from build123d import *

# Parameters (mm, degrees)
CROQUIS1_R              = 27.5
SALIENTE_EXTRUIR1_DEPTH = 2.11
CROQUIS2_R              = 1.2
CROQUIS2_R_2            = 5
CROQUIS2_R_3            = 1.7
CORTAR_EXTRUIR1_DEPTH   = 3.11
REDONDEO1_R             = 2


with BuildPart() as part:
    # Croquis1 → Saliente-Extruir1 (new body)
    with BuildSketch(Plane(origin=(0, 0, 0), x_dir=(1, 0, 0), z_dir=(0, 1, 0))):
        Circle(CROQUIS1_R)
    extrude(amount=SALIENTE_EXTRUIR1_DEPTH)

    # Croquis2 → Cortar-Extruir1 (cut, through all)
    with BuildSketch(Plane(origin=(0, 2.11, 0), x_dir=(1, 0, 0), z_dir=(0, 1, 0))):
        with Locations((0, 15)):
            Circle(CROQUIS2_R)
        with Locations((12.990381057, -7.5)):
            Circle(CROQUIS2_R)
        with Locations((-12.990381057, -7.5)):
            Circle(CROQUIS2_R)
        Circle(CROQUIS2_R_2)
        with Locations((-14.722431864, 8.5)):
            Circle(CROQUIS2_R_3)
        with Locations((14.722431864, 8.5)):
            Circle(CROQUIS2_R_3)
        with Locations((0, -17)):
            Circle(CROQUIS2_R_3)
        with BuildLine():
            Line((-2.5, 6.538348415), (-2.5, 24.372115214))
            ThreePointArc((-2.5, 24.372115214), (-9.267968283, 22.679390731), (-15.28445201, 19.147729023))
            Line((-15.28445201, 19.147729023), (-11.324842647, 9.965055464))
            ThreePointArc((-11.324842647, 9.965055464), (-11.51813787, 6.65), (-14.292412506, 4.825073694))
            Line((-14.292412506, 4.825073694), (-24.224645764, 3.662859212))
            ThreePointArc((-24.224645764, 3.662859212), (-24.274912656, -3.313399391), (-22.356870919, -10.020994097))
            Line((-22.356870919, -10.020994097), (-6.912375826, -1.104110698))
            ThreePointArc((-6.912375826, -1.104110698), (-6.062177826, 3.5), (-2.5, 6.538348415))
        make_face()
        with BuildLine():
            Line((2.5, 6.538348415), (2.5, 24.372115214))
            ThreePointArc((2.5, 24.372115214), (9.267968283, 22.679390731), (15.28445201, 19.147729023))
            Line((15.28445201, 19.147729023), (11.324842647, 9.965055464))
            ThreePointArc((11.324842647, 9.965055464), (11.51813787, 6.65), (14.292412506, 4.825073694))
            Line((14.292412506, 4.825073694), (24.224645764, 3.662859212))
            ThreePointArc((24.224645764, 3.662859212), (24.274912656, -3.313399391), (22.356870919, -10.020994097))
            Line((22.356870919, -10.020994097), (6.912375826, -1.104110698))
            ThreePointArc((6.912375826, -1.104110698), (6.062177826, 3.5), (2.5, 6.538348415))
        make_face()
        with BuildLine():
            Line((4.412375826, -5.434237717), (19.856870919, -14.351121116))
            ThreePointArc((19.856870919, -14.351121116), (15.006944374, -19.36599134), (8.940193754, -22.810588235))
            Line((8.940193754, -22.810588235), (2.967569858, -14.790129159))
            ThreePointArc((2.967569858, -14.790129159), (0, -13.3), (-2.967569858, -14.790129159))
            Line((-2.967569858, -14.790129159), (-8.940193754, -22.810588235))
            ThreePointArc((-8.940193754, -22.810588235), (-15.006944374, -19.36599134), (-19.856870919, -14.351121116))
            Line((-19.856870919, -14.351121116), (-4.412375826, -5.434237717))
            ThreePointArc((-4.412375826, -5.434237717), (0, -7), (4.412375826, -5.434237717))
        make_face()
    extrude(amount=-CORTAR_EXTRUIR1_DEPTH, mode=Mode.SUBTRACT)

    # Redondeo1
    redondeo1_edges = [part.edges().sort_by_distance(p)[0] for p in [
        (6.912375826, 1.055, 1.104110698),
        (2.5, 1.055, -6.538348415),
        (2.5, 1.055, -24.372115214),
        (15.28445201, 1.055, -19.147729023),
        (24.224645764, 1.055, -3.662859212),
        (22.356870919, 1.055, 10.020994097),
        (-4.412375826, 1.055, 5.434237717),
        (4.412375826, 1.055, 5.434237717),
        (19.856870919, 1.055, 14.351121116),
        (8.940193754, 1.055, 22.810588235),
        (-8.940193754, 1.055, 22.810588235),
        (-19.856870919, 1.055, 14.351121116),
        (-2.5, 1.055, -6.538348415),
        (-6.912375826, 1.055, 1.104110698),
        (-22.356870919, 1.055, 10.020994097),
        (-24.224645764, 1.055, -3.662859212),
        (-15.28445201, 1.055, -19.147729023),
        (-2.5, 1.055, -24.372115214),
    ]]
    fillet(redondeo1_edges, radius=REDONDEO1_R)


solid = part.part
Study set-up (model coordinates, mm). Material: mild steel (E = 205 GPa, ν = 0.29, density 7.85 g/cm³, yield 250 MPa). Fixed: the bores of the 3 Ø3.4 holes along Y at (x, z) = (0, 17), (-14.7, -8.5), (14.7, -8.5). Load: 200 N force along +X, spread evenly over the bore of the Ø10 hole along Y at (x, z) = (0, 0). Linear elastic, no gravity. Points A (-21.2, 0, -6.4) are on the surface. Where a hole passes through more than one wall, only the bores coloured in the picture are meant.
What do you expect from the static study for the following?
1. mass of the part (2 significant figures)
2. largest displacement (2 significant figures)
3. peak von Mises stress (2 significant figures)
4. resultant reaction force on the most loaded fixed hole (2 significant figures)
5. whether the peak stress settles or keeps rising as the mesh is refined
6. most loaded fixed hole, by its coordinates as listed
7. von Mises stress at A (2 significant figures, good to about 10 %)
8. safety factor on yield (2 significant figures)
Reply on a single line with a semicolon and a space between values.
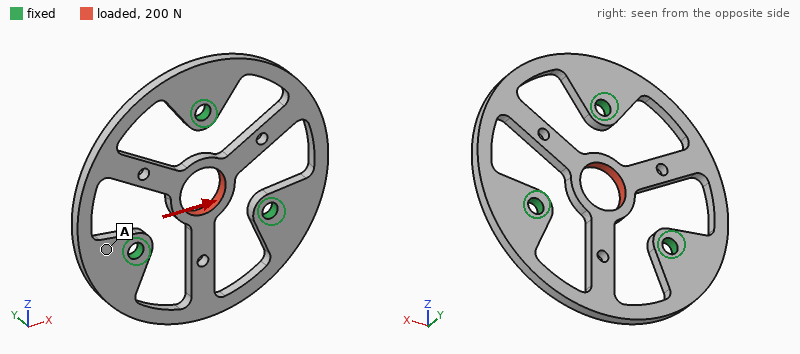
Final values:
19 g; 17 µm; 89 MPa; 130 N; settles; (0, 17); 10 MPa; 2.8
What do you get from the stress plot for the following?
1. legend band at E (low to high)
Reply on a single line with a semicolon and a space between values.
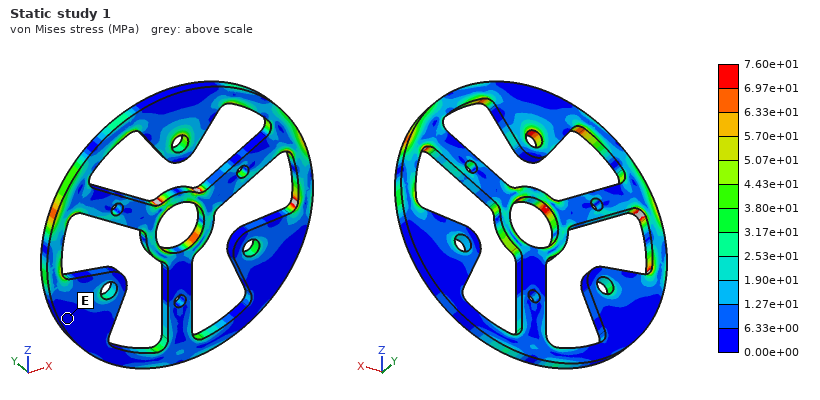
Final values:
0.00e+00 to 6.33e+00 MPa
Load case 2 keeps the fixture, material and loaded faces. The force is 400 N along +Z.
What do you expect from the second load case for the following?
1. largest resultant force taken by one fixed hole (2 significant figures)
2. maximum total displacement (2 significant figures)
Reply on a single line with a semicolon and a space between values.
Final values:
230 N; 36 µm
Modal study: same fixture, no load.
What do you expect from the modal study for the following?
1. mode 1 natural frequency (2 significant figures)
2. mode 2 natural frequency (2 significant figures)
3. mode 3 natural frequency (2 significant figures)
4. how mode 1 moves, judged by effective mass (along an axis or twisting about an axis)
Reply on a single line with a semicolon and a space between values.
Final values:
2700 Hz; 3700 Hz; 3700 Hz; along Y
